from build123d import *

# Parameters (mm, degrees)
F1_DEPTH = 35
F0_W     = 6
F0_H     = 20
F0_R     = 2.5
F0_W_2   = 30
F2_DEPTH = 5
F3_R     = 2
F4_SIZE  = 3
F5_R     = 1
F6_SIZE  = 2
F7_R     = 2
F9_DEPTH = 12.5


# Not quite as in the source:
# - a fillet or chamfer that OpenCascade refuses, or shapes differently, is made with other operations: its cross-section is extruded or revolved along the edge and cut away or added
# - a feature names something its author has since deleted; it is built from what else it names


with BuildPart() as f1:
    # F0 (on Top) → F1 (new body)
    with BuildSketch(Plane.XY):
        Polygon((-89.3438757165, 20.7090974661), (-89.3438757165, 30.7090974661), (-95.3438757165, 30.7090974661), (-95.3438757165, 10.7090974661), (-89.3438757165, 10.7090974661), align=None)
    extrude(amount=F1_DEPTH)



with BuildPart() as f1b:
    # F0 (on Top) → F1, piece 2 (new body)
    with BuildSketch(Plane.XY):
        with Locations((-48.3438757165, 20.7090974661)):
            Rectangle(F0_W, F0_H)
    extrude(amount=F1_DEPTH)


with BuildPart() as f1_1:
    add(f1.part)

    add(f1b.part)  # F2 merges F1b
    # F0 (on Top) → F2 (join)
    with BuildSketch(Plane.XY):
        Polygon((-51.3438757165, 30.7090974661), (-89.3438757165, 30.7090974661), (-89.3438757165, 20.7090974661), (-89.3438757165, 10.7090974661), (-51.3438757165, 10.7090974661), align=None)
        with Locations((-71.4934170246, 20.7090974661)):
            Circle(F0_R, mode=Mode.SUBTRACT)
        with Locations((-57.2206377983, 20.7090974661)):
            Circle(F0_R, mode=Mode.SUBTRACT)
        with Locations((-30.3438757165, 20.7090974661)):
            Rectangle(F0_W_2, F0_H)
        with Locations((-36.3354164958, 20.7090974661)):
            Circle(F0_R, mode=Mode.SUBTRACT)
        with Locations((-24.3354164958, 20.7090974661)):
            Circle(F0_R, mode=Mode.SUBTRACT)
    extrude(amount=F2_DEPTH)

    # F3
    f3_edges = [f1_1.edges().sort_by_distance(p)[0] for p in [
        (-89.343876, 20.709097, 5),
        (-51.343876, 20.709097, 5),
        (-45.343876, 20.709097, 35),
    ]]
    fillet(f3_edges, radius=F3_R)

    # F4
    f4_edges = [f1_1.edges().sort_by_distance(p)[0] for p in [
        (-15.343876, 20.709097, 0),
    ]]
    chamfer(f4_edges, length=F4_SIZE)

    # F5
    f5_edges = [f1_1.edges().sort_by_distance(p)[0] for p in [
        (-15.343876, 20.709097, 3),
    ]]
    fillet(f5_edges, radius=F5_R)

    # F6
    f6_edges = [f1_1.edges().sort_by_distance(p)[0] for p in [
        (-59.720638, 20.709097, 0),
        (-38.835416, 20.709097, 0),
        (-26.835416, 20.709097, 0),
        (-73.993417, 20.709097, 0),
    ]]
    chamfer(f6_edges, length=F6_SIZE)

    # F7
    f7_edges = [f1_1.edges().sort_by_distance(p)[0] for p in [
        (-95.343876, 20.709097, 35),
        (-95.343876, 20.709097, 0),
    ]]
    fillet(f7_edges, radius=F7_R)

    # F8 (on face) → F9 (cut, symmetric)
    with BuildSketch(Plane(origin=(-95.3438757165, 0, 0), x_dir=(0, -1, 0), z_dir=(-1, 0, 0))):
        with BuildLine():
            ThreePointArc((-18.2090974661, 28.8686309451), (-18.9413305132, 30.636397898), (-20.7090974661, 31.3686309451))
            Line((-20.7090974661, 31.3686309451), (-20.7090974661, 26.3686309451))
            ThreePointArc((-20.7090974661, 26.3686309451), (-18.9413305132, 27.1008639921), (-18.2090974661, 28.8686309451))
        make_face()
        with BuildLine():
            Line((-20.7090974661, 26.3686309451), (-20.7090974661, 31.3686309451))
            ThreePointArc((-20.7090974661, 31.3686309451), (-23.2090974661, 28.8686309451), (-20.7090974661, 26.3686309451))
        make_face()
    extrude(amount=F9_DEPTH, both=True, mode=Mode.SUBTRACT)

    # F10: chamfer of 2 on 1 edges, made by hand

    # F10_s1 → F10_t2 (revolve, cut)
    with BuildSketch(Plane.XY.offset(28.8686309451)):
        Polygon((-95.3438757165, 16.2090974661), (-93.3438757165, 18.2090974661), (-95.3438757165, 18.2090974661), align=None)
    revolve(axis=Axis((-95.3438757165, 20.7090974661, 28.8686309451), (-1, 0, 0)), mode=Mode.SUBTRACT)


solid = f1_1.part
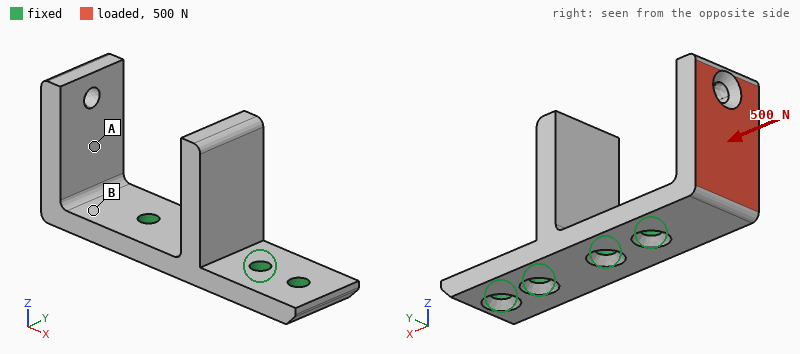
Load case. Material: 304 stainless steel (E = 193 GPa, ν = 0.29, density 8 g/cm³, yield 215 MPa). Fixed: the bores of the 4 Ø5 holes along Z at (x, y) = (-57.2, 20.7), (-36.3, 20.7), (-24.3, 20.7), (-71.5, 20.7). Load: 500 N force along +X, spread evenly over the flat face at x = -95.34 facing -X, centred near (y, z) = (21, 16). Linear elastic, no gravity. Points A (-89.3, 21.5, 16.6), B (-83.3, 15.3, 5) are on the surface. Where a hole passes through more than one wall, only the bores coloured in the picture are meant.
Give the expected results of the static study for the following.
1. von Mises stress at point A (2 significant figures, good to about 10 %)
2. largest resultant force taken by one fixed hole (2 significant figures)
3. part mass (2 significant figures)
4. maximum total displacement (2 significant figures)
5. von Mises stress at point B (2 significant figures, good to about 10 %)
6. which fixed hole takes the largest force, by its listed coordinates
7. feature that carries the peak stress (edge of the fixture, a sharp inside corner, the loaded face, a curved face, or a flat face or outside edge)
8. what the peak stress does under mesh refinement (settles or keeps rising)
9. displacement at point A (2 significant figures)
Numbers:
14 MPa
670 N
120 g
0.14 mm
84 MPa
(-71.5, 20.7)
edge of the fixture
keeps rising
0.061 mm
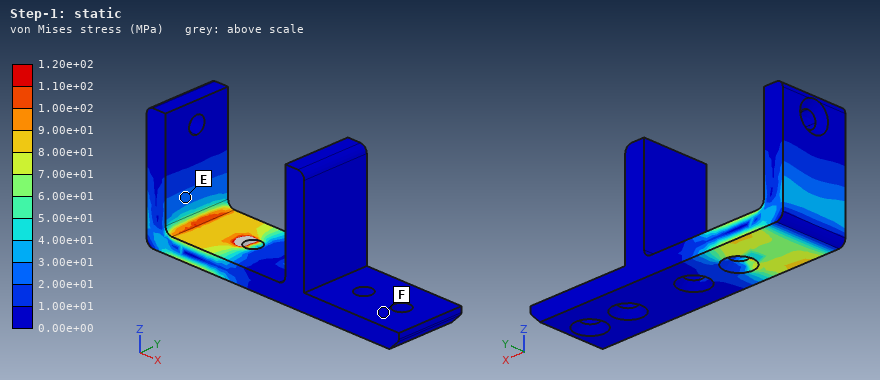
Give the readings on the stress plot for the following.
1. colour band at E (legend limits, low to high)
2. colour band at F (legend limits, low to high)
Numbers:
2.00e+01 to 3.00e+01 MPa
0.00e+00 to 1.00e+01 MPa
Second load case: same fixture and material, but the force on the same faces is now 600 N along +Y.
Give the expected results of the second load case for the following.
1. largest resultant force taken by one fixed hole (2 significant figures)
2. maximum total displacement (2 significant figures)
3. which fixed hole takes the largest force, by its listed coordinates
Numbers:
1.2 kN
0.10 mm
(-71.5, 20.7)
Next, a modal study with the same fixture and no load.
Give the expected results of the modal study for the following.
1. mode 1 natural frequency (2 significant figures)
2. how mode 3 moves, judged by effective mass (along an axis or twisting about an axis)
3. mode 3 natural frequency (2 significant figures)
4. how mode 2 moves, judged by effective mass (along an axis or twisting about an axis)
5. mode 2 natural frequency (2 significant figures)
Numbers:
1700 Hz
along X
4400 Hz
along Y
2500 Hz
